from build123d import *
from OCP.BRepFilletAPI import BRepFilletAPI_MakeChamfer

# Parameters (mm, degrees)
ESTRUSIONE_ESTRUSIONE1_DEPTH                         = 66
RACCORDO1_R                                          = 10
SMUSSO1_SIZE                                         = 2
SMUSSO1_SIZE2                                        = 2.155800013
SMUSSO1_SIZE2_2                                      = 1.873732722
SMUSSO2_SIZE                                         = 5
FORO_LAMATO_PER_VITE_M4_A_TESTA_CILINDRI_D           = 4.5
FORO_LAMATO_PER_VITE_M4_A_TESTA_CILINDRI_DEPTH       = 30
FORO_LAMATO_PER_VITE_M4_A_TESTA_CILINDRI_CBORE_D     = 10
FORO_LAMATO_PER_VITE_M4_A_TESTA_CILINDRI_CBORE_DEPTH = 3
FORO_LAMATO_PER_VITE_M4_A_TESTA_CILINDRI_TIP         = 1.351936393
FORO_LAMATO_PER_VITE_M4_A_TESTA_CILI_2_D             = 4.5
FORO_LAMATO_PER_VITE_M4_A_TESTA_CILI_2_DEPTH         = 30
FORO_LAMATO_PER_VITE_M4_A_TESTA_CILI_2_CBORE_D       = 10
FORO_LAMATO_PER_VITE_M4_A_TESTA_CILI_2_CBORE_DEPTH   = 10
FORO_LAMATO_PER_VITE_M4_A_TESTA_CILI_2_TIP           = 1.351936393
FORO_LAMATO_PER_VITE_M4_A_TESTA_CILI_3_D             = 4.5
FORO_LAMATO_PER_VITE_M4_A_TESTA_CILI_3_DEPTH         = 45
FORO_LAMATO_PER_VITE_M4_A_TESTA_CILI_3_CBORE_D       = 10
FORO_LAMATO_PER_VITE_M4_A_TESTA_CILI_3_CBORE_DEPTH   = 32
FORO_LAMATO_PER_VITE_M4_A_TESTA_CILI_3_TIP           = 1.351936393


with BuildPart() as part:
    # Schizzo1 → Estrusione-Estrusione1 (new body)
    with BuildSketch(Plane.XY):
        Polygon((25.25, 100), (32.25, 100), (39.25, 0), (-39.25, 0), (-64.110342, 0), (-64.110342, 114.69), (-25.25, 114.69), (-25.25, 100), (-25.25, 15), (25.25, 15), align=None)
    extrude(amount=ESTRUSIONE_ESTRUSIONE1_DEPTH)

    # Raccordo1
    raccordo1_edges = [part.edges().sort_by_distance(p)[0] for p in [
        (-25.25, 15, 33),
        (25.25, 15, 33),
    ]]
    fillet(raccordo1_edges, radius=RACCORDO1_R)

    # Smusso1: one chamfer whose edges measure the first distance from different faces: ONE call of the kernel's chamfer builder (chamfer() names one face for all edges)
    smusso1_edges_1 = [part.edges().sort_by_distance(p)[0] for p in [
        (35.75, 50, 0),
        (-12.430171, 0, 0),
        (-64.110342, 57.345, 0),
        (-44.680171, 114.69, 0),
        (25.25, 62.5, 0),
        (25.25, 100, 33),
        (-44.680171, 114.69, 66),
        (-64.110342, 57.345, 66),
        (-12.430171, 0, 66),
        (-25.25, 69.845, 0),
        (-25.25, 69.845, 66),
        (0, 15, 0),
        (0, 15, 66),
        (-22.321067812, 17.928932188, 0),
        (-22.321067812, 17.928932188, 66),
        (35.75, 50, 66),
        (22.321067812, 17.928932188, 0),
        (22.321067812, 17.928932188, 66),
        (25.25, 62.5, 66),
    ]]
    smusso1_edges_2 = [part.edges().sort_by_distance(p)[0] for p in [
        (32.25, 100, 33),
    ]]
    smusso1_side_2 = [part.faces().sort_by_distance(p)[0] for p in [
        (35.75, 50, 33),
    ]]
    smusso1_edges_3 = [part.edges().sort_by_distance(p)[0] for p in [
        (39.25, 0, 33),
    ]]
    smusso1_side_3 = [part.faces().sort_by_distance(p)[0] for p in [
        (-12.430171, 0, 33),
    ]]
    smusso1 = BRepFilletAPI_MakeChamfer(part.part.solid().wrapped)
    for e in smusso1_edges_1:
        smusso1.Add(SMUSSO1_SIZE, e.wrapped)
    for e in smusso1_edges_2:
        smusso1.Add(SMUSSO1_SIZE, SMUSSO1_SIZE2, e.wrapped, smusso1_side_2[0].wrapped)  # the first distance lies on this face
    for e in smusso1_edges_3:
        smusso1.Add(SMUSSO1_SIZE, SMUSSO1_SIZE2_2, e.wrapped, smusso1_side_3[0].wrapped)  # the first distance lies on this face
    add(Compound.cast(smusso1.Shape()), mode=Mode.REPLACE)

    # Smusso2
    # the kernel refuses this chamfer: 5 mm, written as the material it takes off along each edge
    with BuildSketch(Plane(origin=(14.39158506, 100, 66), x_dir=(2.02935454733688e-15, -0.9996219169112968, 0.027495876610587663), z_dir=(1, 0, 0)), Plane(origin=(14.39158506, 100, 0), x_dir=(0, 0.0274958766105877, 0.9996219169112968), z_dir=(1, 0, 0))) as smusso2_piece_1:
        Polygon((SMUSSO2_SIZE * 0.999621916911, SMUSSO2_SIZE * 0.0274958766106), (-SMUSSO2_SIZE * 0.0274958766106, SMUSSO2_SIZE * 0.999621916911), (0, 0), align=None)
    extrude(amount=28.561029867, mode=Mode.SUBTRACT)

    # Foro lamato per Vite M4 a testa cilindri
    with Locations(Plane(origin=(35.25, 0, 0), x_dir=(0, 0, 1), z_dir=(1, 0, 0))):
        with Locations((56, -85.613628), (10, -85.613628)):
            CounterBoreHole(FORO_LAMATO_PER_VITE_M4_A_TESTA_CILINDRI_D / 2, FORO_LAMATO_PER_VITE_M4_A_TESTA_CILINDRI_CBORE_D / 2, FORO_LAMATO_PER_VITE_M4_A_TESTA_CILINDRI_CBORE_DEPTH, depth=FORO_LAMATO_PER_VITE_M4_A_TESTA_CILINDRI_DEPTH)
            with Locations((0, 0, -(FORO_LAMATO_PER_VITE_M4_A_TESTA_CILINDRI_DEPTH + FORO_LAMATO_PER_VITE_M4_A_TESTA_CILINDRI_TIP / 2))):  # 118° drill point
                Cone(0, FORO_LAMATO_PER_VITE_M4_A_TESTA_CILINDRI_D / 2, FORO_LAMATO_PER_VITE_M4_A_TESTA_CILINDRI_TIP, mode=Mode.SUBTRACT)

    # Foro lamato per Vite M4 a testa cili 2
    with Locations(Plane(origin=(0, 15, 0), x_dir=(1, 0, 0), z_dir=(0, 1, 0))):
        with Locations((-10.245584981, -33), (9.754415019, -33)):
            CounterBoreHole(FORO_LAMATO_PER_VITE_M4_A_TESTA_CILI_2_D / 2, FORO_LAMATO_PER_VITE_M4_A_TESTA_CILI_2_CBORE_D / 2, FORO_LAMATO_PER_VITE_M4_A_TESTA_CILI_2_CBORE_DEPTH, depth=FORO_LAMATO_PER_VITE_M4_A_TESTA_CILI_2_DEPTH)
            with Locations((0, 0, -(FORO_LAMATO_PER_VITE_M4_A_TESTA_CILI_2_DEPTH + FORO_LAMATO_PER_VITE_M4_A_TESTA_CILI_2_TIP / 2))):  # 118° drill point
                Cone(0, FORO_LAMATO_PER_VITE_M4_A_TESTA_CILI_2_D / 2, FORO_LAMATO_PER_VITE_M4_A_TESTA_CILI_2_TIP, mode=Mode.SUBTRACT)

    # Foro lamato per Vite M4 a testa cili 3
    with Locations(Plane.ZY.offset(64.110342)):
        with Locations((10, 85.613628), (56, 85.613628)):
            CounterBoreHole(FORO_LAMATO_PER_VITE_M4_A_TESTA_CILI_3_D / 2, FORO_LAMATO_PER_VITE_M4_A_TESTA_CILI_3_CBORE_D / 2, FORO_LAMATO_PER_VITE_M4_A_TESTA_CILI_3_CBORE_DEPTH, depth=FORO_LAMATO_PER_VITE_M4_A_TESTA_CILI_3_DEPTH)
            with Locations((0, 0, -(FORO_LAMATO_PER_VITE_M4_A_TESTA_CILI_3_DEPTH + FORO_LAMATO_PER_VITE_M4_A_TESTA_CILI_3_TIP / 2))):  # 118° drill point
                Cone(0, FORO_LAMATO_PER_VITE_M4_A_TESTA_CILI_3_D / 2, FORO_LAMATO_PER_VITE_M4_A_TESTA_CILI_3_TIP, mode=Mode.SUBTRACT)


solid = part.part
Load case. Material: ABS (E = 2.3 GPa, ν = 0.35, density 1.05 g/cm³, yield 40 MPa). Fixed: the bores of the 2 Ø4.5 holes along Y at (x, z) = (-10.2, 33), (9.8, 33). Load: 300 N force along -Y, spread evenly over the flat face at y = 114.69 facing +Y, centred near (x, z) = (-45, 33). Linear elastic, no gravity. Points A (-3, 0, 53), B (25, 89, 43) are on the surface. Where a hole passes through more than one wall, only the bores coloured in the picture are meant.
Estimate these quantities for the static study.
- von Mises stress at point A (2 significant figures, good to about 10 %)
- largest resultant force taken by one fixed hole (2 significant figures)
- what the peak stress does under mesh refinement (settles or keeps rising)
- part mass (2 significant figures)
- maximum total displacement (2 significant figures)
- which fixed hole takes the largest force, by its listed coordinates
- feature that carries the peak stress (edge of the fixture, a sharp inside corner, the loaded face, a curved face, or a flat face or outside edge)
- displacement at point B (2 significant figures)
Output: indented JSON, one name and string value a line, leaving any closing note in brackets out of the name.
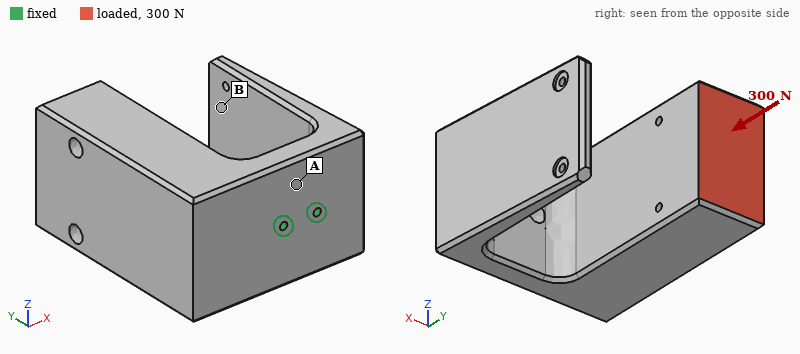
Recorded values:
{
  "von Mises stress at point A": "2.0 MPa",
  "largest resultant force taken by one fixed hole": "730 N",
  "what the peak stress does under mesh refinement": "keeps rising",
  "part mass": "430 g",
  "maximum total displacement": "1.1 mm",
  "which fixed hole takes the largest force, by its listed coordinates": "(-10.2, 33)",
  "feature that carries the peak stress": "edge of the fixture",
  "displacement at point B": "0.33 mm"
}
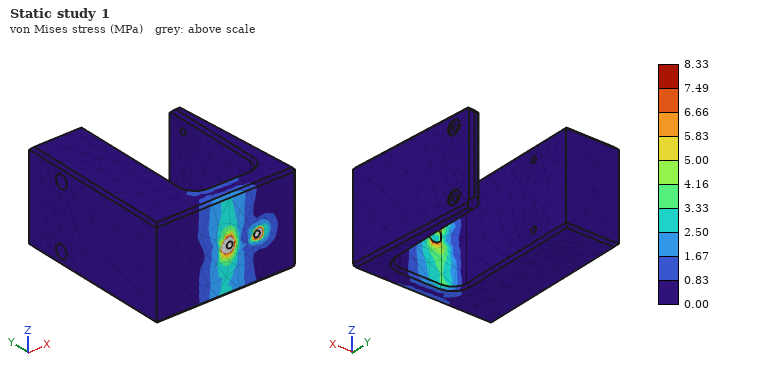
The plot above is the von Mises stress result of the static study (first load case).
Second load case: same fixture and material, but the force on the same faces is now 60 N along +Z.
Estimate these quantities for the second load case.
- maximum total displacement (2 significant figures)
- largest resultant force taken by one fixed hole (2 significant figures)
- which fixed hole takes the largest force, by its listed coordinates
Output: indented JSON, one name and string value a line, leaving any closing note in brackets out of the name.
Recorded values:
{
  "maximum total displacement": "1.9 mm",
  "largest resultant force taken by one fixed hole": "150 N",
  "which fixed hole takes the largest force, by its listed coordinates": "(-10.2, 33)"
}
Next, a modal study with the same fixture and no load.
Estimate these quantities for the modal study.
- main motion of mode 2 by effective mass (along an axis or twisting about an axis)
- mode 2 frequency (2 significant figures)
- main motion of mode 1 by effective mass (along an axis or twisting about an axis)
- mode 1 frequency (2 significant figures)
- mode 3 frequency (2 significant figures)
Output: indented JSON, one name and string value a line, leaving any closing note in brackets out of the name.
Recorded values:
{
  "main motion of mode 2 by effective mass": "along X",
  "mode 2 frequency": "130 Hz",
  "main motion of mode 1 by effective mass": "along Z",
  "mode 1 frequency": "83 Hz",
  "mode 3 frequency": "330 Hz"
}
